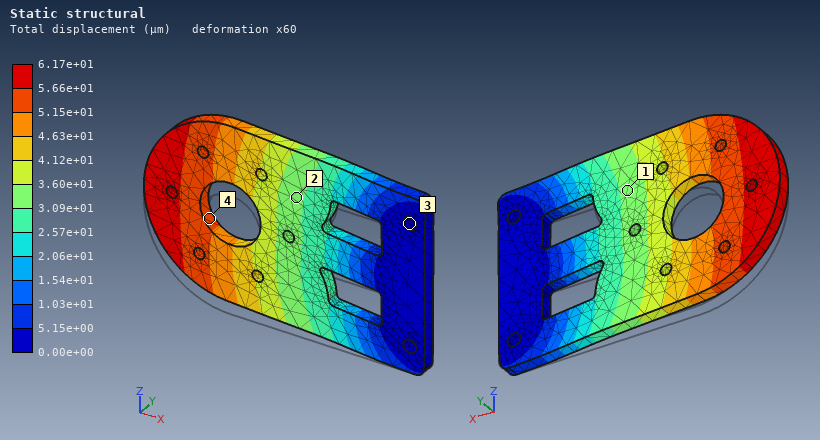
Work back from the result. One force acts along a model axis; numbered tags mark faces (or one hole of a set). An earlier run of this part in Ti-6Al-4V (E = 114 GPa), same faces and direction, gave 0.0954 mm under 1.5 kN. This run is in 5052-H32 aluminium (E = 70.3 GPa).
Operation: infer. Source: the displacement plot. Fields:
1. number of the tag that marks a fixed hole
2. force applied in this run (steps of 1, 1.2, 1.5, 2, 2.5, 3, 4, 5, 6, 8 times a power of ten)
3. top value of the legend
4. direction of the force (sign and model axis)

3
600 N
6.17e+01 µm
+Z
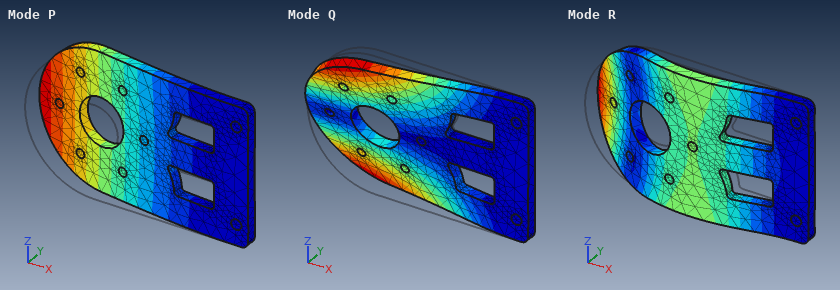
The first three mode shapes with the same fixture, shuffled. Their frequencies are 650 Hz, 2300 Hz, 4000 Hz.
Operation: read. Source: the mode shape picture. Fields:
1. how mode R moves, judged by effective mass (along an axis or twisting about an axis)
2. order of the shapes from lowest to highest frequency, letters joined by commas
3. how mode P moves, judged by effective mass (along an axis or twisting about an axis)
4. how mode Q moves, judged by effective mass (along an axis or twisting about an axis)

along Y
P, Q, R
along Y
twisting about X
